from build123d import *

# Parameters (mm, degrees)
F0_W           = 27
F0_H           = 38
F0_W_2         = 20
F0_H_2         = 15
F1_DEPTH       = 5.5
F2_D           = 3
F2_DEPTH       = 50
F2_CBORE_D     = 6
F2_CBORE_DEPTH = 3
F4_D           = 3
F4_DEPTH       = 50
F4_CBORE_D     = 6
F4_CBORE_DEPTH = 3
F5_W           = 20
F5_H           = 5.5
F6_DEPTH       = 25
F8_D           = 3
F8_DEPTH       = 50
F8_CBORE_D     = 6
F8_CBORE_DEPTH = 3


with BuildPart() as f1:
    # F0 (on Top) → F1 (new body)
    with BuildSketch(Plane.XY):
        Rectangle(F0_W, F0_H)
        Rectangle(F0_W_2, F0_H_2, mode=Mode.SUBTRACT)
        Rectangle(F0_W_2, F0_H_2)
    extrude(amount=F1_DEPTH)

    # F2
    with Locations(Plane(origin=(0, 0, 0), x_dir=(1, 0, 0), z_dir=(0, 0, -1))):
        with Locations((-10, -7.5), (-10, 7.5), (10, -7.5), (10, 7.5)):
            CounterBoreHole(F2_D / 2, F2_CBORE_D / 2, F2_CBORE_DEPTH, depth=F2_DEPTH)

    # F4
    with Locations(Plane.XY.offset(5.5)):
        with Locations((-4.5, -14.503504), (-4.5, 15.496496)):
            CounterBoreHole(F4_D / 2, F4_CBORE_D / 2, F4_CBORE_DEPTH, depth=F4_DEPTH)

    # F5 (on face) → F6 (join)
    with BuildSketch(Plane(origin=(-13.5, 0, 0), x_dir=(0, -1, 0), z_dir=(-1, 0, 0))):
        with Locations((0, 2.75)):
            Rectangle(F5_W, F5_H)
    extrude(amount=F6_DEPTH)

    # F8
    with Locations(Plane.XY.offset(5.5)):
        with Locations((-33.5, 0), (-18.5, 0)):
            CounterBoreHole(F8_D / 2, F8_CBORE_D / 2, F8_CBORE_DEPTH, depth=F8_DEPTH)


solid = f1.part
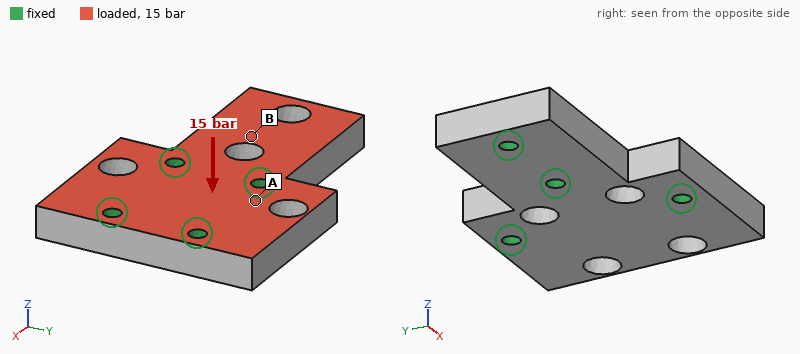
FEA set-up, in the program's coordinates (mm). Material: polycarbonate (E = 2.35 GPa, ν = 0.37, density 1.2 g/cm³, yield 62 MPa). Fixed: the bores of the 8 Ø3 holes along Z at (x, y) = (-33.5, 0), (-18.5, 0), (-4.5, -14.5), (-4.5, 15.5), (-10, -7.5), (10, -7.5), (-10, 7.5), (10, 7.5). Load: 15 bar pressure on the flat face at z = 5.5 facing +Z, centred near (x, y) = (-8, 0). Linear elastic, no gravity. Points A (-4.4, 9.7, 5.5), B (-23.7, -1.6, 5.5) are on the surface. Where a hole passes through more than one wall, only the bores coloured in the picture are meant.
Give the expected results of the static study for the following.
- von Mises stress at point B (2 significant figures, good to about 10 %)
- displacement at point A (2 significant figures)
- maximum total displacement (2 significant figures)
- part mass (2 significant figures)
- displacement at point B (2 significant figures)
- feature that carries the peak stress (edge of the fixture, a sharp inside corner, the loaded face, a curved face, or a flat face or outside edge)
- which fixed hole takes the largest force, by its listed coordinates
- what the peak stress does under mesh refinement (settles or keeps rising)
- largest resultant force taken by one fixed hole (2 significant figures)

9.5 MPa
0.031 mm
0.16 mm
9.1 g
0.046 mm
edge of the fixture
(-33.5, 0)
keeps rising
340 N
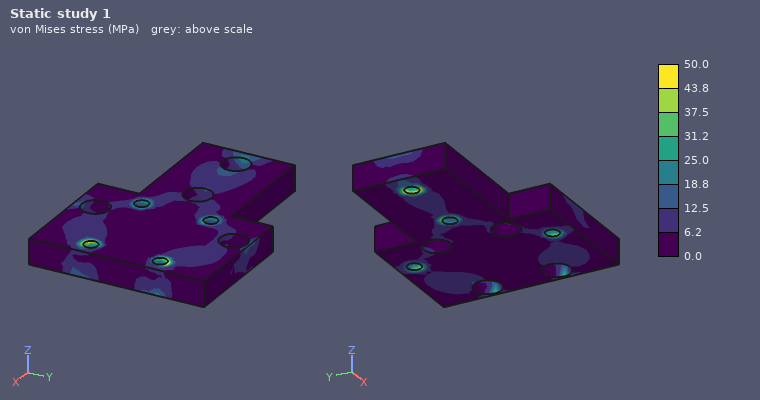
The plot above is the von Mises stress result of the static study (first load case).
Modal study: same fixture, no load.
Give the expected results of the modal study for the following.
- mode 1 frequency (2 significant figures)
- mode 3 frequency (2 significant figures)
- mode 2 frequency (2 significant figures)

5600 Hz
7600 Hz
7500 Hz
